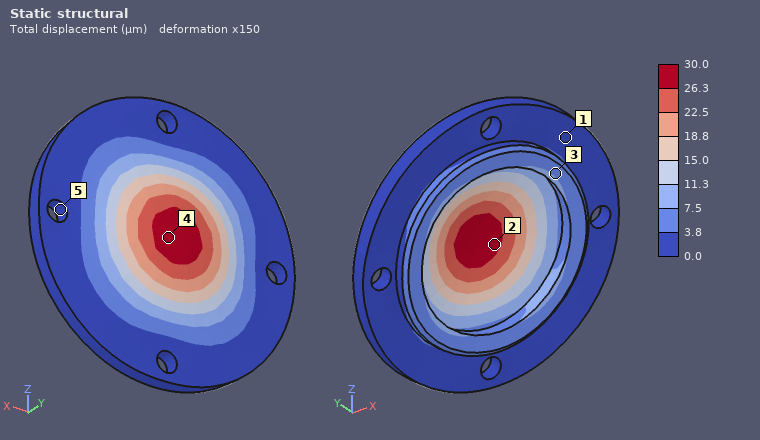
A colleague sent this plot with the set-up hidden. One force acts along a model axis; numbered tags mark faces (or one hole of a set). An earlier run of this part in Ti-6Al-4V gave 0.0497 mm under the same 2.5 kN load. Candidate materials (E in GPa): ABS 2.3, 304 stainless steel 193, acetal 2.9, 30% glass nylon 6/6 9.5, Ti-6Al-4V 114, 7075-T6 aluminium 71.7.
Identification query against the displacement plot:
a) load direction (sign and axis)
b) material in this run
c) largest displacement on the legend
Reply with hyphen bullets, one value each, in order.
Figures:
- +Y
- 304 stainless steel
- 30.0 µm
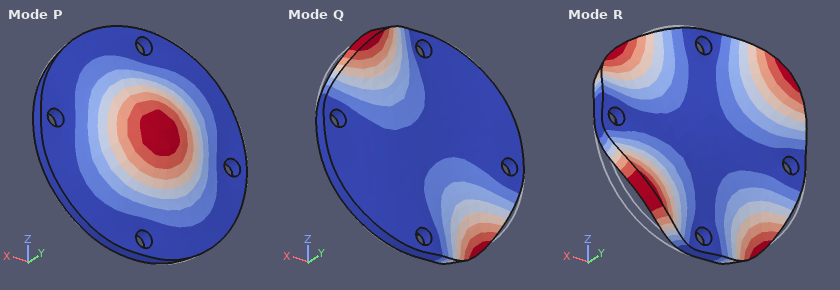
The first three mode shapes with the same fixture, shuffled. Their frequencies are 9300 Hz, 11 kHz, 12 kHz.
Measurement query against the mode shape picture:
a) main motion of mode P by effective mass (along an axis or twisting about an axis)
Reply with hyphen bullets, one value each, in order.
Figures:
- along Y
